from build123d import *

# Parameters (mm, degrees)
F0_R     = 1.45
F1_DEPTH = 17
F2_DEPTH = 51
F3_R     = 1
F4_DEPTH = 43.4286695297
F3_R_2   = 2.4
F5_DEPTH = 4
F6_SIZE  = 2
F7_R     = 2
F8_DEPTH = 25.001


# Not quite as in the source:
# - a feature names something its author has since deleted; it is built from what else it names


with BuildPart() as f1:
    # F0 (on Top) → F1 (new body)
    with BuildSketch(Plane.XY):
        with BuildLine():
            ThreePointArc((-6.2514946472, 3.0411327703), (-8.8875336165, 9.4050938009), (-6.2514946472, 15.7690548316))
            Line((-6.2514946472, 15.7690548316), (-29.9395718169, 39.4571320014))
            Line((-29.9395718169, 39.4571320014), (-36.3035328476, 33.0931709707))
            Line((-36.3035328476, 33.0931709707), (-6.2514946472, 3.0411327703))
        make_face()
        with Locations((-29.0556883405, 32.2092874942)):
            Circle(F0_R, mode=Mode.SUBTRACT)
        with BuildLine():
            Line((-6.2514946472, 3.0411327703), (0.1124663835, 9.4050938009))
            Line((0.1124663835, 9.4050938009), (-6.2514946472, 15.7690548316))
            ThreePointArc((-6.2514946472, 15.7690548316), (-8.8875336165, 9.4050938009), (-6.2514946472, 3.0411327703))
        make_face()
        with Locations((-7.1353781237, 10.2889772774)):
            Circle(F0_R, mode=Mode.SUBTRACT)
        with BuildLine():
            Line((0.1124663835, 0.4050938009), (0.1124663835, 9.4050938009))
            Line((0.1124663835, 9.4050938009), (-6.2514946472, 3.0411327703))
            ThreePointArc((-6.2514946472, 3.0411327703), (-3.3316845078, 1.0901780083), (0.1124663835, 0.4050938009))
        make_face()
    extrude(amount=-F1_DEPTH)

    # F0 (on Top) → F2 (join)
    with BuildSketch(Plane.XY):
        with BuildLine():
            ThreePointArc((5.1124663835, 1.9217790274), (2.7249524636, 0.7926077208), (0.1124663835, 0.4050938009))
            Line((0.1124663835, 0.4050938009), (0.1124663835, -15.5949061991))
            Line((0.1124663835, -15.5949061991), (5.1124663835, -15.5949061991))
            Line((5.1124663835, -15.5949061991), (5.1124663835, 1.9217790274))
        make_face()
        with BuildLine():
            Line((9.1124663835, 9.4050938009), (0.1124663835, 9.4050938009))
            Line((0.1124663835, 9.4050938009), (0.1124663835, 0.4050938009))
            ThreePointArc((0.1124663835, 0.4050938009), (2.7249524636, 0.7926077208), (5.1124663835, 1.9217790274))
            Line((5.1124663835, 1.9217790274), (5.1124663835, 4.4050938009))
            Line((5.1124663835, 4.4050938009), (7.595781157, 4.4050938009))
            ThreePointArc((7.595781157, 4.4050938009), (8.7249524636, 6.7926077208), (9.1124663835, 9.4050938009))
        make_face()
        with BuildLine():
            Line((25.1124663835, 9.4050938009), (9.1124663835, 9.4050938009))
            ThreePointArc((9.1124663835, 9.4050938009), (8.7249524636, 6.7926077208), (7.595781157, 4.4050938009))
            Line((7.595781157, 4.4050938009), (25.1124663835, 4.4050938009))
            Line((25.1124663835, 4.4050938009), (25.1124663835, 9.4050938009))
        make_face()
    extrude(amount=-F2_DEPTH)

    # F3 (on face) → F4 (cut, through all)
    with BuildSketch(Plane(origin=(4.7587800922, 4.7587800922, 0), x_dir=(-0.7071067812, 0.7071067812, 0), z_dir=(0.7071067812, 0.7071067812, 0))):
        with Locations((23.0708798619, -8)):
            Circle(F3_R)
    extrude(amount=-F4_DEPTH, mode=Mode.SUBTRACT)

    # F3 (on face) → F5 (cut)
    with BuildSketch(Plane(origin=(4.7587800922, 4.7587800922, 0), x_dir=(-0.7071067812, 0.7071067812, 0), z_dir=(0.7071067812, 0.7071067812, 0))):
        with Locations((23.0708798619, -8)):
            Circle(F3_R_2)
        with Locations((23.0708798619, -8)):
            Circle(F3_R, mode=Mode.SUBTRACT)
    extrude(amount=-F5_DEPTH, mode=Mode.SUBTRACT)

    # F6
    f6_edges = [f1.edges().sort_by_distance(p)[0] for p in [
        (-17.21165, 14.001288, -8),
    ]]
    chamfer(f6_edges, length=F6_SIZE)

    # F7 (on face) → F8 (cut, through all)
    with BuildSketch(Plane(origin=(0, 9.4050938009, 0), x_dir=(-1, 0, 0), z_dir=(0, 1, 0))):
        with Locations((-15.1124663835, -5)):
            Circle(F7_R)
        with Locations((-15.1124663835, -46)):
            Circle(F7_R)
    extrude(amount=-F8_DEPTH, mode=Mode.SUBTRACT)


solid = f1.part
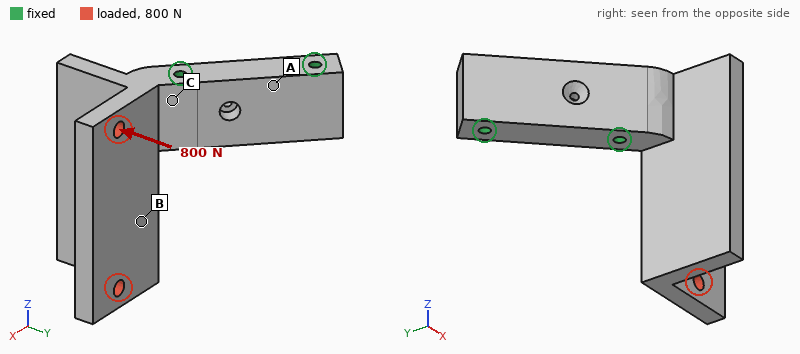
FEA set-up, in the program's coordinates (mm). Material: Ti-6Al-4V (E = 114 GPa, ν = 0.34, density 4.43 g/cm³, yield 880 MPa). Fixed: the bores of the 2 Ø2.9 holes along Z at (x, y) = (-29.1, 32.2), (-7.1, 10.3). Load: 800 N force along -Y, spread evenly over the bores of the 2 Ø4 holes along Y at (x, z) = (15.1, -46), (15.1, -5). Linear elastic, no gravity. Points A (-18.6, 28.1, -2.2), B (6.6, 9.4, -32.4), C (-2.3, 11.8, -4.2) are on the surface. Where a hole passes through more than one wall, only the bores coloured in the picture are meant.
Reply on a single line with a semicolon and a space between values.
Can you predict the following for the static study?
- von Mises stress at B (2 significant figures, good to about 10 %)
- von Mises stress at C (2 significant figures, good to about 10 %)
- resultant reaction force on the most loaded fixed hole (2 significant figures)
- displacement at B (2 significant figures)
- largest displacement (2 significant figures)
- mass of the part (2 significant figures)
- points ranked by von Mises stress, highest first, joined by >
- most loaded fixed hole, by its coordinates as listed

28 MPa; 58 MPa; 980 N; 0.054 mm; 0.17 mm; 80 g; C > B > A; (-7.1, 10.3)
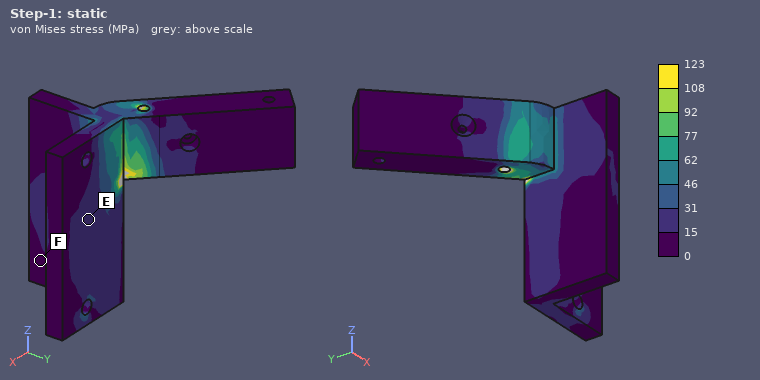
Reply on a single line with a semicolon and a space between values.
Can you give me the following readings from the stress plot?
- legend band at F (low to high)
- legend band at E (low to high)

0 to 15 MPa; 15 to 31 MPa
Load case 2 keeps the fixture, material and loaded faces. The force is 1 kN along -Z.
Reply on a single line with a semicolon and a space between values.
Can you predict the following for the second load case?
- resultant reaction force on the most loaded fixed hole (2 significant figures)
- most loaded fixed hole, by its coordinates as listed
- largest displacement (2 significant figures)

1.0 kN; (-7.1, 10.3); 55 µm
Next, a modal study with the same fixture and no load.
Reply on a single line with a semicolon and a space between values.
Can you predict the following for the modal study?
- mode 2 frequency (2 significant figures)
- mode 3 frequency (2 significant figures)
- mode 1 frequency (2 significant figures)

3800 Hz; 4500 Hz; 2400 Hz
